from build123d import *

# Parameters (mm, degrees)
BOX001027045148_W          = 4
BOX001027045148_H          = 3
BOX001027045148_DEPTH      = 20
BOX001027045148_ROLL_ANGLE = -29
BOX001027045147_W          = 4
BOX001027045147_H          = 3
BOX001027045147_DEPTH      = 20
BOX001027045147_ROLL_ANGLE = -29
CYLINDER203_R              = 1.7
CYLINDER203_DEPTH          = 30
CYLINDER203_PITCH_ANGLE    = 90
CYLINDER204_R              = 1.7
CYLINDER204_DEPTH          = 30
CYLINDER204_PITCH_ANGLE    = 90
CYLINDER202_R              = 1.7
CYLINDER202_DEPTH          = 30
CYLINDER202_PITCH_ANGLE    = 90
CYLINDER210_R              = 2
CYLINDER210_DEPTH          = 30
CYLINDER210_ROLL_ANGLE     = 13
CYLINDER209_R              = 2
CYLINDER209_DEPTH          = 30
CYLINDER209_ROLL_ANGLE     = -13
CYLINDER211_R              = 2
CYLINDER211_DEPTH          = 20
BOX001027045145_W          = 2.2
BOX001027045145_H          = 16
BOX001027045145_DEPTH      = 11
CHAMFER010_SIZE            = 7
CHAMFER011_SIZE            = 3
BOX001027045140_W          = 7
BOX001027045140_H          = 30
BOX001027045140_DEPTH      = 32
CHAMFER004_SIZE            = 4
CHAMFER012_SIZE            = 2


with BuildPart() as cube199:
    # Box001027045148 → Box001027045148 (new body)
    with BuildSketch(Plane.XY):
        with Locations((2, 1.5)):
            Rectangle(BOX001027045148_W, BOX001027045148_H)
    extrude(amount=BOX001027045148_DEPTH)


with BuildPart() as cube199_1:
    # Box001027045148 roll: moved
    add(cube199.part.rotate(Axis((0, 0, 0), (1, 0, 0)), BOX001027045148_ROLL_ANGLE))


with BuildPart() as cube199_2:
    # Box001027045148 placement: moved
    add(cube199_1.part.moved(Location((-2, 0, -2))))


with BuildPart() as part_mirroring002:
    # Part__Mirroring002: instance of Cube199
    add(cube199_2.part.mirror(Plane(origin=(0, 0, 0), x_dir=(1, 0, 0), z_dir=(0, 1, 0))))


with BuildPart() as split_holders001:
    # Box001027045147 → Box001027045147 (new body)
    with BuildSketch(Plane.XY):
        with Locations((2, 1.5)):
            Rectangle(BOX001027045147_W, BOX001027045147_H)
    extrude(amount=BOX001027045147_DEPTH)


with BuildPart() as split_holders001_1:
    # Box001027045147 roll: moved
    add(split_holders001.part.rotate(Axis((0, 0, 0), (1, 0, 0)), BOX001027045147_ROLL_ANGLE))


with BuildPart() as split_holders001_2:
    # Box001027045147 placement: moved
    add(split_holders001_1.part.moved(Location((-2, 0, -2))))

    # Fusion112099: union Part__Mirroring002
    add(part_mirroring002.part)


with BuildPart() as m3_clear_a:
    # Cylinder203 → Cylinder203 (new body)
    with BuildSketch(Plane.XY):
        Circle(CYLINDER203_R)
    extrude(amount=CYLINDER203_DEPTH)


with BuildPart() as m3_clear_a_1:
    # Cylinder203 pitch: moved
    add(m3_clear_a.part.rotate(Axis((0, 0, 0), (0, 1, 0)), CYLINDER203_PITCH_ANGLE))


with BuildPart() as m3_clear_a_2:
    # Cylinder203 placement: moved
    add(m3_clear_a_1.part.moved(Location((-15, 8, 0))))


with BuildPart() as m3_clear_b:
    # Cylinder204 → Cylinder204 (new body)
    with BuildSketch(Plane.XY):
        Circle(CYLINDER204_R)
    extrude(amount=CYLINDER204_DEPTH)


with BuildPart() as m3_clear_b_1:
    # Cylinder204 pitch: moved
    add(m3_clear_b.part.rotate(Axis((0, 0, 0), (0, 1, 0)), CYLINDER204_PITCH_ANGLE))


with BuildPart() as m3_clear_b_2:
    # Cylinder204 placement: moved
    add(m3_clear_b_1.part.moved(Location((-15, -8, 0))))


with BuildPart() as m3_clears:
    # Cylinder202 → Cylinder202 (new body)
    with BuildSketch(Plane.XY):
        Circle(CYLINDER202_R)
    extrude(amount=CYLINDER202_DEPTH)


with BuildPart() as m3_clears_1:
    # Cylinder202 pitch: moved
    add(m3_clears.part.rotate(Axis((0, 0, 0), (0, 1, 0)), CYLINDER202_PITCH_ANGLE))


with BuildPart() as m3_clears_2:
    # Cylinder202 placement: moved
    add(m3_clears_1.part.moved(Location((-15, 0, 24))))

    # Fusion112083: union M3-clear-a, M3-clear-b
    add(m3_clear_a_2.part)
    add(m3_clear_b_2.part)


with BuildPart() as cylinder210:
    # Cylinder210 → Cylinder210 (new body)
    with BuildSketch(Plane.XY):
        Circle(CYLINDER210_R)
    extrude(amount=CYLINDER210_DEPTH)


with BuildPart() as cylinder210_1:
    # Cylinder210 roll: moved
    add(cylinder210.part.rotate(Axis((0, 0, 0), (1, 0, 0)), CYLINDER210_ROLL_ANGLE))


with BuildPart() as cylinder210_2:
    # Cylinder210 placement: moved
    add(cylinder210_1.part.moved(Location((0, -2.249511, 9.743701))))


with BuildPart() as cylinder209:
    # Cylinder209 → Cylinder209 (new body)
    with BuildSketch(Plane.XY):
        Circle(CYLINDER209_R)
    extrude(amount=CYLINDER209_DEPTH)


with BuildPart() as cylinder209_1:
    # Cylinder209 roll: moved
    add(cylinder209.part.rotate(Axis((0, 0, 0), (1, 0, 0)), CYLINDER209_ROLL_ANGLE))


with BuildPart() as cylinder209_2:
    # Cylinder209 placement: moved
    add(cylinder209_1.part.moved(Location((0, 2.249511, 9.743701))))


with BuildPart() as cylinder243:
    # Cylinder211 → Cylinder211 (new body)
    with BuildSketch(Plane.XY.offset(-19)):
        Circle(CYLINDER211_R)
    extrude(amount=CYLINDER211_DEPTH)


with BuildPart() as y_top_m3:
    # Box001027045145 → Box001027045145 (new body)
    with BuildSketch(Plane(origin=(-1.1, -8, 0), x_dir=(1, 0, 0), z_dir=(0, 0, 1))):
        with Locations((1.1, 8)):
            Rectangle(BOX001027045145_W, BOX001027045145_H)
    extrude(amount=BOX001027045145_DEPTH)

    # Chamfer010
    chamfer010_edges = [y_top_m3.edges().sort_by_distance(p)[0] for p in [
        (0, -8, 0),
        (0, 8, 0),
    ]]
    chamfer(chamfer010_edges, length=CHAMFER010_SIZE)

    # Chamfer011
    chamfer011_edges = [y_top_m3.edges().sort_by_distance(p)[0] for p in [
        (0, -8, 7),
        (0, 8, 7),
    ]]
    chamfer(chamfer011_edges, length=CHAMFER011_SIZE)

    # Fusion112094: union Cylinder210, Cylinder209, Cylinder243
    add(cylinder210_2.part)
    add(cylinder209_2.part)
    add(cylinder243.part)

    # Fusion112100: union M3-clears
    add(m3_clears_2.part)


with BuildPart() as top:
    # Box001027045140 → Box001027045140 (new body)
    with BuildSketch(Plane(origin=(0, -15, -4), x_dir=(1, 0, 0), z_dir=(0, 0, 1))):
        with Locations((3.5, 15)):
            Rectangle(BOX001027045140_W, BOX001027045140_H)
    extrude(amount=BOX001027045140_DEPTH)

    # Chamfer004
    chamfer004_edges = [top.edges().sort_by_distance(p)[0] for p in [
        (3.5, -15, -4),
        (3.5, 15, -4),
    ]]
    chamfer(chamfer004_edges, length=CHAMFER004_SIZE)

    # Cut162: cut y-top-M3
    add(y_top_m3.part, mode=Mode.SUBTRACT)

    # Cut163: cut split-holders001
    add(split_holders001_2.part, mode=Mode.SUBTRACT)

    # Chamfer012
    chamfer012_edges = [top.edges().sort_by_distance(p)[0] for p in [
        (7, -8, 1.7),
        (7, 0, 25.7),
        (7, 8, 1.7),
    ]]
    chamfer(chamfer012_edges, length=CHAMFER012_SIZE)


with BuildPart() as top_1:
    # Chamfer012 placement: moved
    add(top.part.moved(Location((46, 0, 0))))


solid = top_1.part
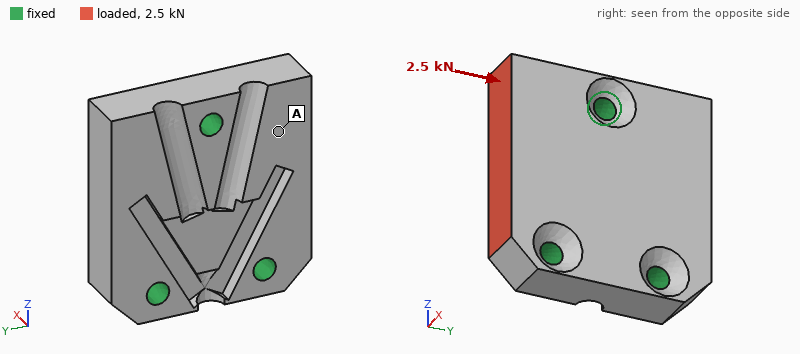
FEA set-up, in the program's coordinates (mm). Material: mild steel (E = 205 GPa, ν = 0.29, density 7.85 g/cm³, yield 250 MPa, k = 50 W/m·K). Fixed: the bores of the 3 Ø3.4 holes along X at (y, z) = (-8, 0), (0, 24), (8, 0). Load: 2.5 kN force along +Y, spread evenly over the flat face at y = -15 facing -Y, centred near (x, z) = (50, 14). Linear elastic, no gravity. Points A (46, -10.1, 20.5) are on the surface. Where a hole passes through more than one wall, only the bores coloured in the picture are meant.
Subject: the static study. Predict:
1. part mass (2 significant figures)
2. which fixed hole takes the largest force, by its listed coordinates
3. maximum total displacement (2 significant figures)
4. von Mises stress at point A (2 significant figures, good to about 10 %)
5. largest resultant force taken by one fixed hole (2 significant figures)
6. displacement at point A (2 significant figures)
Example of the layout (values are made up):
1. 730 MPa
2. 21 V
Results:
1. 45 g
2. (0, 24)
3. 2.1 µm
4. 11 MPa
5. 1.4 kN
6. 1.6 µm
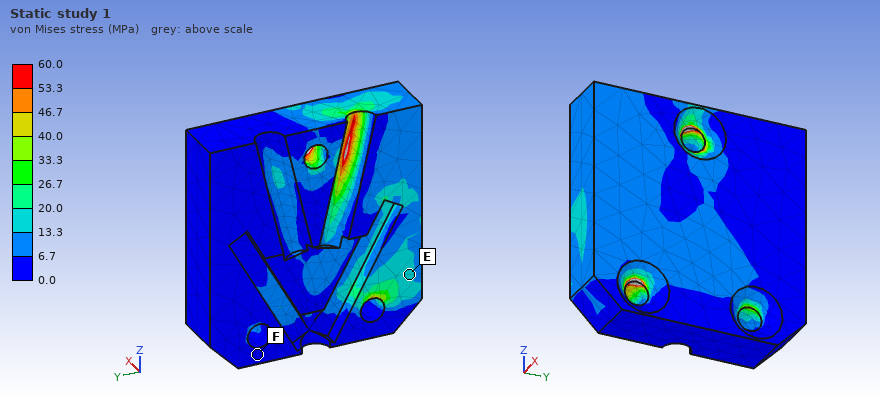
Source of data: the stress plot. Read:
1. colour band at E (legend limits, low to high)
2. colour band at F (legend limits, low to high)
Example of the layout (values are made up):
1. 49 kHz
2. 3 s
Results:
1. 13.3 to 20.0 MPa
2. 0.0 to 6.7 MPa
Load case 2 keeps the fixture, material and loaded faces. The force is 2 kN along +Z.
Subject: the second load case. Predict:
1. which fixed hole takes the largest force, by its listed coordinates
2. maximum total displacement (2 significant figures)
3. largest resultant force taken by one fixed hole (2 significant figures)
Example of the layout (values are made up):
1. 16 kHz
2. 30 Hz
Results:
1. (-8, 0)
2. 3.7 µm
3. 1.5 kN
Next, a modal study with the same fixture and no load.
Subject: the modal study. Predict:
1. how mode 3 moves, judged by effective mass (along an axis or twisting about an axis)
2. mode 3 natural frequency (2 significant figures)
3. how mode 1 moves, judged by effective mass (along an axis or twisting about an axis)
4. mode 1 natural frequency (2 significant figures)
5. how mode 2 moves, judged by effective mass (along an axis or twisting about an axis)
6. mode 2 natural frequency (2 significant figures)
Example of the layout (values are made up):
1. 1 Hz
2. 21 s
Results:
1. along X
2. 36 kHz
3. twisting about Z
4. 18 kHz
5. along X
6. 21 kHz
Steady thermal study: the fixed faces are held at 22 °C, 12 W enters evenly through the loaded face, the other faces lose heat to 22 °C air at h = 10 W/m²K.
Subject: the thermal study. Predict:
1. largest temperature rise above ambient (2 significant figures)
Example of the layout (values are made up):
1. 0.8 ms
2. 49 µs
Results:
1. 21 K
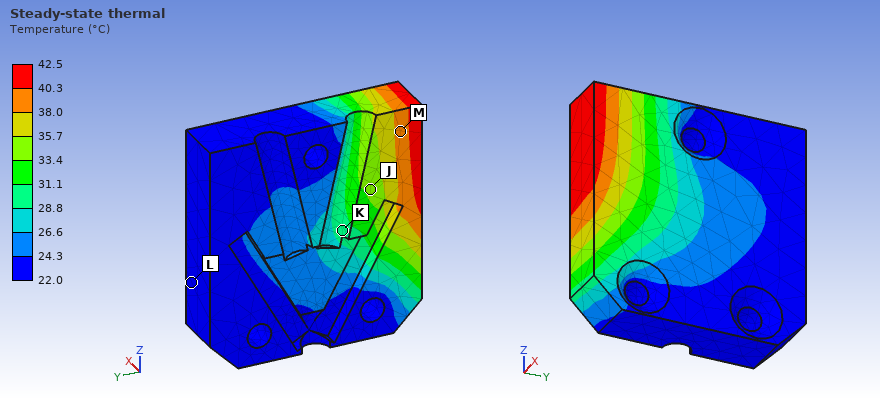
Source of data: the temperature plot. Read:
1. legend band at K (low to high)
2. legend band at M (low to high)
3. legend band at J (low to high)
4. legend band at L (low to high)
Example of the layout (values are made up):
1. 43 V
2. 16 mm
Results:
1. 28.8 to 31.1 °C
2. 38.0 to 40.3 °C
3. 33.4 to 35.7 °C
4. 22.0 to 24.3 °C
